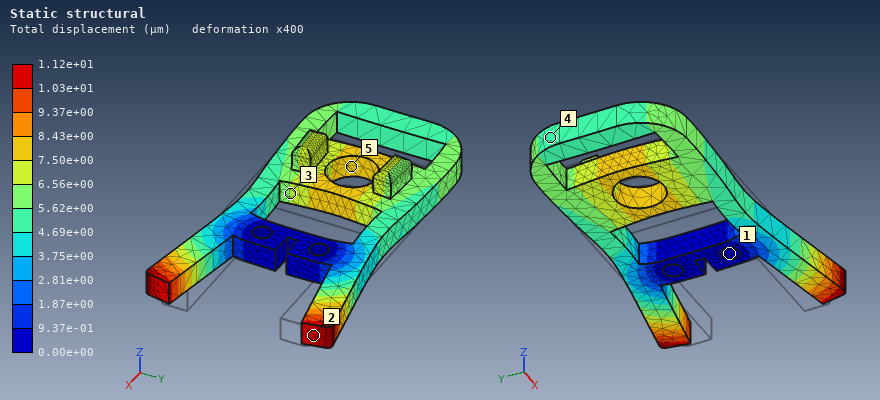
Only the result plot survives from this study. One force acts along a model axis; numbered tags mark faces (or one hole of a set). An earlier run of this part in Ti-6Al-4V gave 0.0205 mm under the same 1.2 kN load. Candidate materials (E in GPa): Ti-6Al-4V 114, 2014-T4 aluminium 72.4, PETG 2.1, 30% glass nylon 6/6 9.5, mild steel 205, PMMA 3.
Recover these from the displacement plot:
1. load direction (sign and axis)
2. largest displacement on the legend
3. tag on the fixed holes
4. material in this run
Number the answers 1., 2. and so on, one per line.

1. -X
2. 1.12e+01 µm
3. 1
4. mild steel
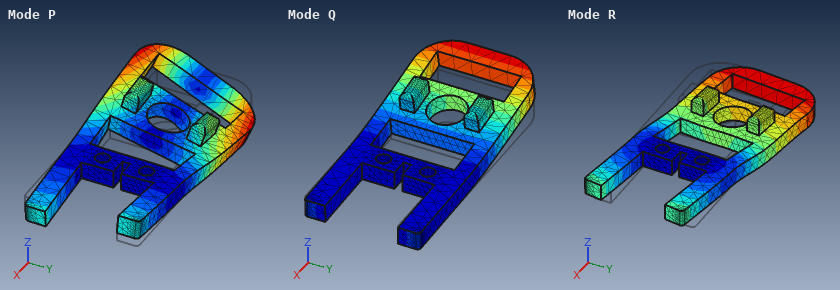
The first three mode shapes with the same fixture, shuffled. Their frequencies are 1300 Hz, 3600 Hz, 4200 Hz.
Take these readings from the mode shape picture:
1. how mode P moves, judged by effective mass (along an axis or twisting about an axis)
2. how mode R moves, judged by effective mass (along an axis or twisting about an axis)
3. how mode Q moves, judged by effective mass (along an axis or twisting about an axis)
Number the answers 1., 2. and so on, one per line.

1. twisting about X
2. along Y
3. along Z
